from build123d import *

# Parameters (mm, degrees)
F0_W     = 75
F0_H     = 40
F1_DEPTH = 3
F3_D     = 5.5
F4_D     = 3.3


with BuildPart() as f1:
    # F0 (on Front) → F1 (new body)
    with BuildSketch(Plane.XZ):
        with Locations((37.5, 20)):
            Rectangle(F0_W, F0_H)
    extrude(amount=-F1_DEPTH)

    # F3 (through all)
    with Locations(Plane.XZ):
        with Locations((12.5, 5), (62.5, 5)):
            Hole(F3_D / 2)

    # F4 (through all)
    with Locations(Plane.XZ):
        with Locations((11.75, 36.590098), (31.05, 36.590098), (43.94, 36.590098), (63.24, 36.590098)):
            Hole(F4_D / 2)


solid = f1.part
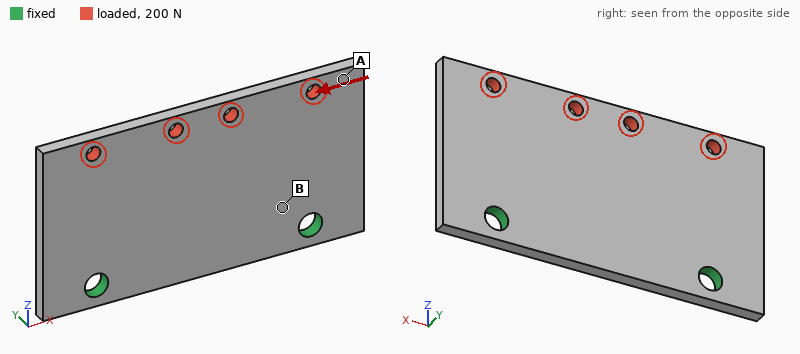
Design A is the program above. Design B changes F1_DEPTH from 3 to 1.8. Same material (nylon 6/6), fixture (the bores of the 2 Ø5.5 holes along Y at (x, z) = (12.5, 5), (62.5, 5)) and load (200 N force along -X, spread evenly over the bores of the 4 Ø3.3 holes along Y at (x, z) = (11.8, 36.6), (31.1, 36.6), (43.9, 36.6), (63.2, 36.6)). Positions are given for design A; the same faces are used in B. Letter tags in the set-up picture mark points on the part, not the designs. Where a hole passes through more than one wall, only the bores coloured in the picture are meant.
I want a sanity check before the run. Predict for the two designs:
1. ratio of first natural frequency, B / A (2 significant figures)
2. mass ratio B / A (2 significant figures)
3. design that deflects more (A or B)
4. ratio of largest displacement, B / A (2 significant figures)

0.62
0.60
B
1.7
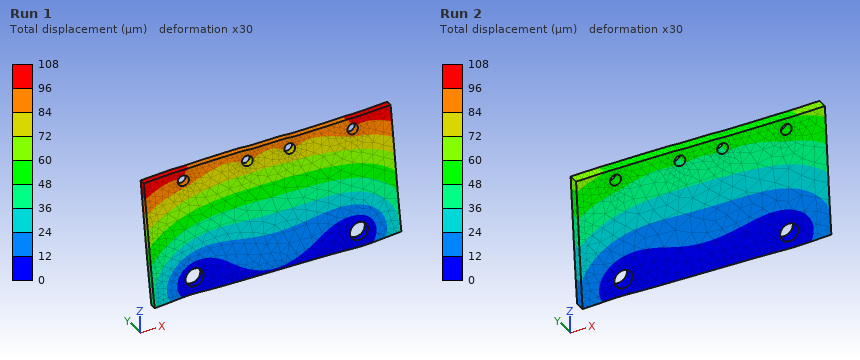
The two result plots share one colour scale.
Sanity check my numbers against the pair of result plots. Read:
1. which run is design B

Run 1
